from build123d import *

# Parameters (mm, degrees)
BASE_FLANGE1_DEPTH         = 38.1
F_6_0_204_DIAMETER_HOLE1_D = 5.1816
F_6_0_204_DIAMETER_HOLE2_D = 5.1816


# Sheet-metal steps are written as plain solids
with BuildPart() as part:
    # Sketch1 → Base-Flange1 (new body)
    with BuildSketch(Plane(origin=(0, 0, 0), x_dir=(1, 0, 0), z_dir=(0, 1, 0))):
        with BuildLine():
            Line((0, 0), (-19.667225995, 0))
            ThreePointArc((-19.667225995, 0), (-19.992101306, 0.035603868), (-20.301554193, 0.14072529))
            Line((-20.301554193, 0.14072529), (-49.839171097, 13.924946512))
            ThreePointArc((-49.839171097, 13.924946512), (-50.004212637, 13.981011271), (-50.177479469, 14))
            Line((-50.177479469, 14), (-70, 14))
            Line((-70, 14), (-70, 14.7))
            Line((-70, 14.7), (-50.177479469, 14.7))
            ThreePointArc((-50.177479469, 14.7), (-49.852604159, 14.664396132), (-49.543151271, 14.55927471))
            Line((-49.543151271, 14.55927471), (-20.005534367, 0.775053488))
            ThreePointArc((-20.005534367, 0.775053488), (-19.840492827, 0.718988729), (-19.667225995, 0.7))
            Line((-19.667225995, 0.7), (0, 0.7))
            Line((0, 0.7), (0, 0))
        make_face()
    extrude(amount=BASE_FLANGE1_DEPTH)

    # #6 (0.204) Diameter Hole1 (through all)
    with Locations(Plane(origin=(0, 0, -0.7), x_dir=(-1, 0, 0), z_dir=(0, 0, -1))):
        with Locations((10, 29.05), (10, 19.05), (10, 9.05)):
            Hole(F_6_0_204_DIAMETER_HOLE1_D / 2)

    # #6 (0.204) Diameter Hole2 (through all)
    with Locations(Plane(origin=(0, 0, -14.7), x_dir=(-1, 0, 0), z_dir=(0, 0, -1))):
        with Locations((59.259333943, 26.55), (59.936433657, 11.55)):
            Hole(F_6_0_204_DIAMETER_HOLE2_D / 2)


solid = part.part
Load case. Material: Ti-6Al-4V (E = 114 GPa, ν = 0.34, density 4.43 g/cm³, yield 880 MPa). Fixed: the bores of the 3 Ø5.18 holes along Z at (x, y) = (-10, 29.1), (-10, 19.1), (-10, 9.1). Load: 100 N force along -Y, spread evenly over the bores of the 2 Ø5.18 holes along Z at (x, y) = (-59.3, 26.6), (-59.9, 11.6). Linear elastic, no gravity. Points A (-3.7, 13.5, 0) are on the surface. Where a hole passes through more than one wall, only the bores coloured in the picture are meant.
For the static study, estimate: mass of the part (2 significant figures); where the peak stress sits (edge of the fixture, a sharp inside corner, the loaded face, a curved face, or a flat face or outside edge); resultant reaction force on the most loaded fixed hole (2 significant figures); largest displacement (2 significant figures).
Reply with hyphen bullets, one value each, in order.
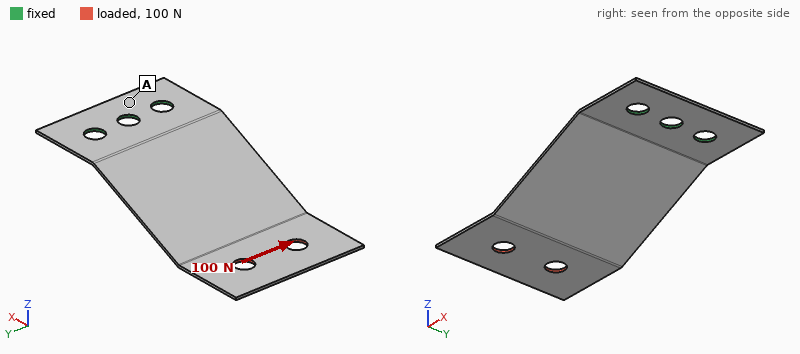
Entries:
- 8.3 g
- a flat face or outside edge
- 220 N
- 0.93 mm
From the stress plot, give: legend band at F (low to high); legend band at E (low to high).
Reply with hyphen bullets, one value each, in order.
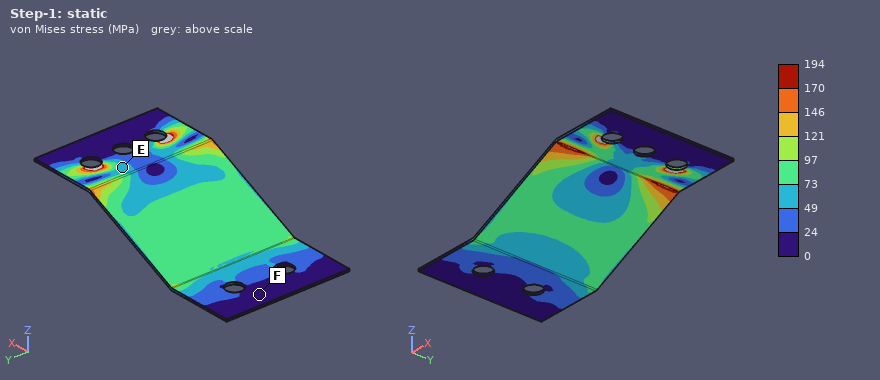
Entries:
- 0 to 24 MPa
- 49 to 73 MPa
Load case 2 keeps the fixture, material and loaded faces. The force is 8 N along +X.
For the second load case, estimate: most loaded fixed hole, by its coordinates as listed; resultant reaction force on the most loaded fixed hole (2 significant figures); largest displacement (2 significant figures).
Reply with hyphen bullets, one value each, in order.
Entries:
- (-10, 19.1)
- 3.7 N
- 0.94 mm
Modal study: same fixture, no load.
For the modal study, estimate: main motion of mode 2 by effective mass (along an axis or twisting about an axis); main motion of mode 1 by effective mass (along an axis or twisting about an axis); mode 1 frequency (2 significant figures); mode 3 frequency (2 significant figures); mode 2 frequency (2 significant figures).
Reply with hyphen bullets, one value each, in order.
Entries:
- twisting about X
- along Z
- 170 Hz
- 990 Hz
- 540 Hz
